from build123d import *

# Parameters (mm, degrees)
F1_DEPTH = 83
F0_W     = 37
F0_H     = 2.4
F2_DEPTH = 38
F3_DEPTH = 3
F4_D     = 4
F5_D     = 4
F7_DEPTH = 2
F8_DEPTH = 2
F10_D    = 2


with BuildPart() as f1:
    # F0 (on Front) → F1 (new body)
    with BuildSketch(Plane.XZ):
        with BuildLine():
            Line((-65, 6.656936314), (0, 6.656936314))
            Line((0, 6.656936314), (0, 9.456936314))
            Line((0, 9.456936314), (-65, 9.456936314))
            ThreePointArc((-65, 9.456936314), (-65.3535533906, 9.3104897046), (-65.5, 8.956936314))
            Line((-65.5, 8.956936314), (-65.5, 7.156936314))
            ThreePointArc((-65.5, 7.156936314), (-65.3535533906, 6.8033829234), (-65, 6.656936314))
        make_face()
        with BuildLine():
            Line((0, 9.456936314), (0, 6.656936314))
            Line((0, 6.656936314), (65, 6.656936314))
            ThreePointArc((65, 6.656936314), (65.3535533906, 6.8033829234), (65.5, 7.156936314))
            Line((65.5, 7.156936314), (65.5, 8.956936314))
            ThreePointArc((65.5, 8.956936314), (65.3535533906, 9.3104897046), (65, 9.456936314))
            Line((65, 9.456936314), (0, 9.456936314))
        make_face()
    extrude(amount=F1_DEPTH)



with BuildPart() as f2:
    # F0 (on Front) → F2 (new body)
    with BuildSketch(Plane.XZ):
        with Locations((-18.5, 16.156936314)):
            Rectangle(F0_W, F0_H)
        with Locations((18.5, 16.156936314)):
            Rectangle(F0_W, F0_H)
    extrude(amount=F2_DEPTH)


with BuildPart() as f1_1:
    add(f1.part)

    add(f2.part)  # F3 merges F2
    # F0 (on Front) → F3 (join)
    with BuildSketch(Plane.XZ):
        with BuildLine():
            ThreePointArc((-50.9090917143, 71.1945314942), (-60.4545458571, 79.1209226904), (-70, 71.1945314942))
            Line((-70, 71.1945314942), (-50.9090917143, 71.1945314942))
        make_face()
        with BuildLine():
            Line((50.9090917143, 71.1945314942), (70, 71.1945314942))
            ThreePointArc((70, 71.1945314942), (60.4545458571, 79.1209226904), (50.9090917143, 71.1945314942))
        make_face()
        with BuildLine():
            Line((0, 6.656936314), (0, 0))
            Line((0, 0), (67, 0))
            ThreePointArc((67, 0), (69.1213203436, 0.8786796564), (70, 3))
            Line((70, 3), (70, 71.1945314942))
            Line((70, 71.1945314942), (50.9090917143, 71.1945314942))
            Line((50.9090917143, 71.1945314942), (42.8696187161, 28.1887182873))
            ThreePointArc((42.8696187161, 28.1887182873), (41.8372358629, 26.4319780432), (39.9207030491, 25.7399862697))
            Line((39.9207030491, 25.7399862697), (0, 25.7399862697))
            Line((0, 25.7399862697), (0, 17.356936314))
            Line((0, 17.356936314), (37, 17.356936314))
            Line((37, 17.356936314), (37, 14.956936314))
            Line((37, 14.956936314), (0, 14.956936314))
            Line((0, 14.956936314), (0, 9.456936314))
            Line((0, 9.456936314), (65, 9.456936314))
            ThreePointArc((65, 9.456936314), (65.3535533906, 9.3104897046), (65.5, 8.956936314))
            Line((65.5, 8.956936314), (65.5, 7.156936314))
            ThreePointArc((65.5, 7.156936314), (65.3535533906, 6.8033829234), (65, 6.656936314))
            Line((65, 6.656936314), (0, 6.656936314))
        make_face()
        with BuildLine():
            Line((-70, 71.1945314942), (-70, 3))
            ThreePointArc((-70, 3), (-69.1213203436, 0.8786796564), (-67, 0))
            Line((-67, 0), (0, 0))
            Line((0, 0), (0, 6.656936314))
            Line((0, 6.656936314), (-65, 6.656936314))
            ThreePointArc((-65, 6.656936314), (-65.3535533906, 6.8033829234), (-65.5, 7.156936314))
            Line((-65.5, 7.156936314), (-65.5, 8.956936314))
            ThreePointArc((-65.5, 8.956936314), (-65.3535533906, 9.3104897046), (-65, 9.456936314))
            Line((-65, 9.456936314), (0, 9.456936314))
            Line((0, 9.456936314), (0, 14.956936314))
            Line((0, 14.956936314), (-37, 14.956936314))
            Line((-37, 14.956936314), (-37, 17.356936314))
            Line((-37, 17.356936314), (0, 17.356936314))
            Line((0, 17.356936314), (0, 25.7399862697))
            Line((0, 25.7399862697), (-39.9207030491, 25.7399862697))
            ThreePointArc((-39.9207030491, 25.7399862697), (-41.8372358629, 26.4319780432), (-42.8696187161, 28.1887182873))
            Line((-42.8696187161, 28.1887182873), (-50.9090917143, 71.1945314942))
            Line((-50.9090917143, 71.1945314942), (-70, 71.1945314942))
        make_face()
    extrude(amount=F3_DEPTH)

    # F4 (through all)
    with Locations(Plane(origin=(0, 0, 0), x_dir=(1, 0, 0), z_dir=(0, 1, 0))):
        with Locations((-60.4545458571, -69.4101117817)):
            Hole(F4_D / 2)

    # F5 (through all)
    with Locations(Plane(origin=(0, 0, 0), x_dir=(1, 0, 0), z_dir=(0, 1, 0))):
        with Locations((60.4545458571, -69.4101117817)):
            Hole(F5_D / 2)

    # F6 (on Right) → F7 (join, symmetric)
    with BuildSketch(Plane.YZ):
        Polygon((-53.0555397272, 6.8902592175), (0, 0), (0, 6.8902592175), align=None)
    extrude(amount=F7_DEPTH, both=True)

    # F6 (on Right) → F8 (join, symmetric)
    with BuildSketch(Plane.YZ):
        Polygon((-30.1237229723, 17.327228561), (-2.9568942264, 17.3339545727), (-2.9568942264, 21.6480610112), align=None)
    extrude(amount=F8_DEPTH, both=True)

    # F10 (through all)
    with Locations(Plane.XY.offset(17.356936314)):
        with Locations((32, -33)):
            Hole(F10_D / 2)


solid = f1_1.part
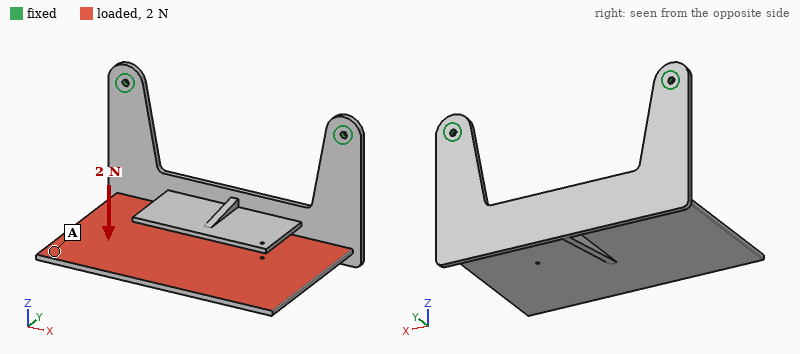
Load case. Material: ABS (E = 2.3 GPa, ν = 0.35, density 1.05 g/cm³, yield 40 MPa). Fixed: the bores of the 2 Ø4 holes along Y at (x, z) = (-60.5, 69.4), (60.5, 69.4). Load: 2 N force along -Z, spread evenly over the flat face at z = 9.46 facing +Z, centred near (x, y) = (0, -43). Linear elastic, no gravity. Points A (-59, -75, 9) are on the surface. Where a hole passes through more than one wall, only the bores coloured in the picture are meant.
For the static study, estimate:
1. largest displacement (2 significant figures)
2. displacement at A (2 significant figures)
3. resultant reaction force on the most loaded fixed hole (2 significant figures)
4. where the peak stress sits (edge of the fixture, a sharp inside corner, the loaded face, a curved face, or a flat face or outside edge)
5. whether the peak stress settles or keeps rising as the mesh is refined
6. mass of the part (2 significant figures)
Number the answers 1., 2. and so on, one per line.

1. 1.8 mm
2. 1.6 mm
3. 1.1 N
4. edge of the fixture
5. keeps rising
6. 57 g
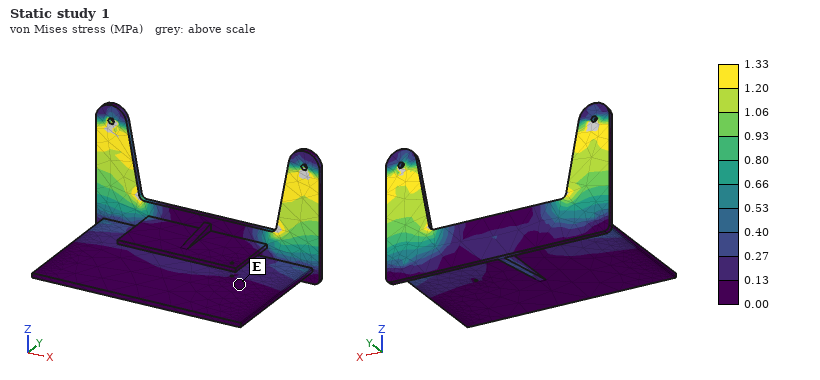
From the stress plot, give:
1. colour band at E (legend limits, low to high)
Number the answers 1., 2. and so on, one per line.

1. 0.00 to 0.13 MPa
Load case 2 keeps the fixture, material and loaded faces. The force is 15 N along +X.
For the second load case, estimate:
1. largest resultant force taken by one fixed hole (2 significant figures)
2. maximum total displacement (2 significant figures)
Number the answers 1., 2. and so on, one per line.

1. 11 N
2. 1.9 mm
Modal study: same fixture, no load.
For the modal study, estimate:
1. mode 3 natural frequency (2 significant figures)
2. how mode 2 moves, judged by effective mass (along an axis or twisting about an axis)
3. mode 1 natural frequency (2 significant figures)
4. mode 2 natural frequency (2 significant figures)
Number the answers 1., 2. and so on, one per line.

1. 97 Hz
2. along X
3. 29 Hz
4. 80 Hz
